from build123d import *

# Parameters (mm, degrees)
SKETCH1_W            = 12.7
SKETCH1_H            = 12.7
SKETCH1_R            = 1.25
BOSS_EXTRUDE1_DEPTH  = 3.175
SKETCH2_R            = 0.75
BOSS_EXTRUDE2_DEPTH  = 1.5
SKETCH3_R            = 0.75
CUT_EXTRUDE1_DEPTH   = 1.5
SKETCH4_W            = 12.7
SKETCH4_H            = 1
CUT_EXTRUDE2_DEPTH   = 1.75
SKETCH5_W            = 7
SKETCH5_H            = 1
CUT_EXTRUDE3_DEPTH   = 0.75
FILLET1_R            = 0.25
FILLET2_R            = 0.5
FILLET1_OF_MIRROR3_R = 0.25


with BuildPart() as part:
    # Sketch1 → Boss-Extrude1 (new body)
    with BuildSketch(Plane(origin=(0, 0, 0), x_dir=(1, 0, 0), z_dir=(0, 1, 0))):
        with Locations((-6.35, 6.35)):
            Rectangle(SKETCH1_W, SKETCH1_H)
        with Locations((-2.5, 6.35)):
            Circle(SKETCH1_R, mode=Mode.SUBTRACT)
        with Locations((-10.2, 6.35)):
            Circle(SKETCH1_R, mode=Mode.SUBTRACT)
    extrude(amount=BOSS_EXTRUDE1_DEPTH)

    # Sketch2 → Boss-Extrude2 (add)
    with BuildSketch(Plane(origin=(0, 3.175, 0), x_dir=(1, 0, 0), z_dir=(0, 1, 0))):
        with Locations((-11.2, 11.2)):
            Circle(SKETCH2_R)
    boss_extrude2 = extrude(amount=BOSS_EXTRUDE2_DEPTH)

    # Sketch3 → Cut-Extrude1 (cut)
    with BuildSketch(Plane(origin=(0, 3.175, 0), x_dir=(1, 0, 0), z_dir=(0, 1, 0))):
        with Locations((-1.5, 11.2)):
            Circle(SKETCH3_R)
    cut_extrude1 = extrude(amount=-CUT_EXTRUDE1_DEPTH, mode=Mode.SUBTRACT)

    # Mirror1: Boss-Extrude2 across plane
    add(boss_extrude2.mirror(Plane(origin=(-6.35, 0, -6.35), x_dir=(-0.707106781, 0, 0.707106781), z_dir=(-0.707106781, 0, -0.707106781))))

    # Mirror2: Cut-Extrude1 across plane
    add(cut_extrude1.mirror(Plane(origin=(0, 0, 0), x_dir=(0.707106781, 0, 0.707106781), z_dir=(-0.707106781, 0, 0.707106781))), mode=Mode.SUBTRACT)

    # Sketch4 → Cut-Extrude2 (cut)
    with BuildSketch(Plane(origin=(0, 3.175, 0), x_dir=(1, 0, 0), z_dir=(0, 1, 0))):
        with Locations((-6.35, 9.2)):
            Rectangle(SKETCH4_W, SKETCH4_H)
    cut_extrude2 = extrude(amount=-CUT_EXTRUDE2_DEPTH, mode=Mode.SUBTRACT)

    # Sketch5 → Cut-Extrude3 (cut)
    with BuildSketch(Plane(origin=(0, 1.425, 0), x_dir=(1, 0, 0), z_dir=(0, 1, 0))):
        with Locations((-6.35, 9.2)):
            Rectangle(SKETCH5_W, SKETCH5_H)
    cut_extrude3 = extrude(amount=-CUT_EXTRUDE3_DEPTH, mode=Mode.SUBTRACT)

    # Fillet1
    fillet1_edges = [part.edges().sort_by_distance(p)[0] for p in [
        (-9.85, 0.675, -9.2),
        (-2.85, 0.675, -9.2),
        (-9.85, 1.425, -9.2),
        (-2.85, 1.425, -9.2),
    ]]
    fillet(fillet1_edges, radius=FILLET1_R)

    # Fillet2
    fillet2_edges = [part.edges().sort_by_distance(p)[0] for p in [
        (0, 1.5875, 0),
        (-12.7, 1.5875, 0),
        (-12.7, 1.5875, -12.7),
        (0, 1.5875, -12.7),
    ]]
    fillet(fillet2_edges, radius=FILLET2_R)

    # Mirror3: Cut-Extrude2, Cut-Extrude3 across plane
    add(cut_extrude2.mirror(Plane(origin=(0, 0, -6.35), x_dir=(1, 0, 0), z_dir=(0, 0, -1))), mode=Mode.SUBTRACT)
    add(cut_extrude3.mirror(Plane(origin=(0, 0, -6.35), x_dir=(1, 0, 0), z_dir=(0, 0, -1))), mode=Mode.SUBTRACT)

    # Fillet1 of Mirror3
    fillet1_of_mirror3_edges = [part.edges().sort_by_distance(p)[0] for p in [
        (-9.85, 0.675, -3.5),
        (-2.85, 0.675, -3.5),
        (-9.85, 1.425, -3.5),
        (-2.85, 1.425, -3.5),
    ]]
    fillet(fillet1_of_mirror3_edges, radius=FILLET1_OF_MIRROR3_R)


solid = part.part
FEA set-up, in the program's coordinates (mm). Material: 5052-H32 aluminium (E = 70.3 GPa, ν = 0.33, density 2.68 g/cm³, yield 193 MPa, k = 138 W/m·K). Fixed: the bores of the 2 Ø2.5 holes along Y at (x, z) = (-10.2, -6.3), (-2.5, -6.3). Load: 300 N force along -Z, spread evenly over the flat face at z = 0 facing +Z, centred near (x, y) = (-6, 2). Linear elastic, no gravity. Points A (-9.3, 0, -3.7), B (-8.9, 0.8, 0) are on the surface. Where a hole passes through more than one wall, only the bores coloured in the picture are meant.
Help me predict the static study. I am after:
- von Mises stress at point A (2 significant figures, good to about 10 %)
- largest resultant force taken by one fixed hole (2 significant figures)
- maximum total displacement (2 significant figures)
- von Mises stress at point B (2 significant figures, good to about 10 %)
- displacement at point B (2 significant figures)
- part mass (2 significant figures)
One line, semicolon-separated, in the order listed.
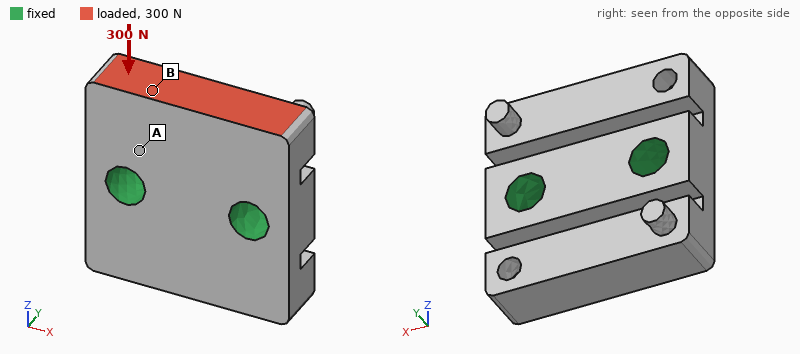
64 MPa; 150 N; 26 µm; 14 MPa; 19 µm; 1.1 g
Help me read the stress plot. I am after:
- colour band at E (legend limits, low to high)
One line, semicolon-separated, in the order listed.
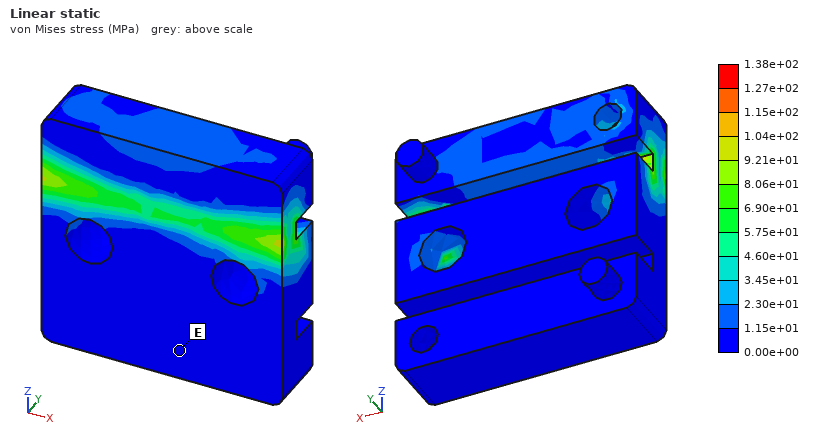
0.00e+00 to 1.15e+01 MPa
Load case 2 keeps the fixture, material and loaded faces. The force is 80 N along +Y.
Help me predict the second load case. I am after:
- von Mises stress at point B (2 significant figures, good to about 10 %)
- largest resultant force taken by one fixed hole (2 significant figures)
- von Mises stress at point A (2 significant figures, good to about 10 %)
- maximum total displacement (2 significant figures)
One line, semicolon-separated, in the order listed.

12 MPa; 40 N; 87 MPa; 25 µm
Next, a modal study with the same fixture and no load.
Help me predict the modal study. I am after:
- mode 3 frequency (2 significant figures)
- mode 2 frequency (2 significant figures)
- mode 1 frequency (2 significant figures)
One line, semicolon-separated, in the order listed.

52 kHz; 24 kHz; 24 kHz
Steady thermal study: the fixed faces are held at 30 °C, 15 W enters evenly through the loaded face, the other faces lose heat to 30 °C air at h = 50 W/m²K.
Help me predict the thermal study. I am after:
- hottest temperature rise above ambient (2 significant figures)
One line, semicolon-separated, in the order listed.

31 K
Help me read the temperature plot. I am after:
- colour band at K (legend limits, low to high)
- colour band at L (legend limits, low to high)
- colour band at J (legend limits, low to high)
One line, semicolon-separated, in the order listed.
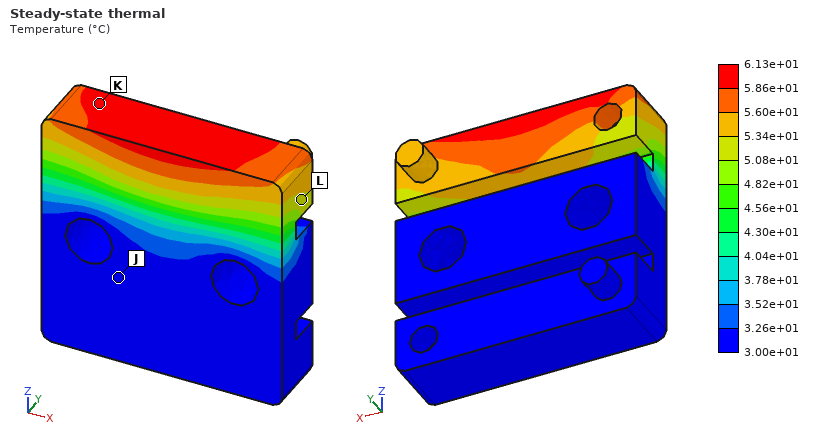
5.86e+01 to 6.13e+01 °C; 5.08e+01 to 5.34e+01 °C; 3.00e+01 to 3.26e+01 °C
